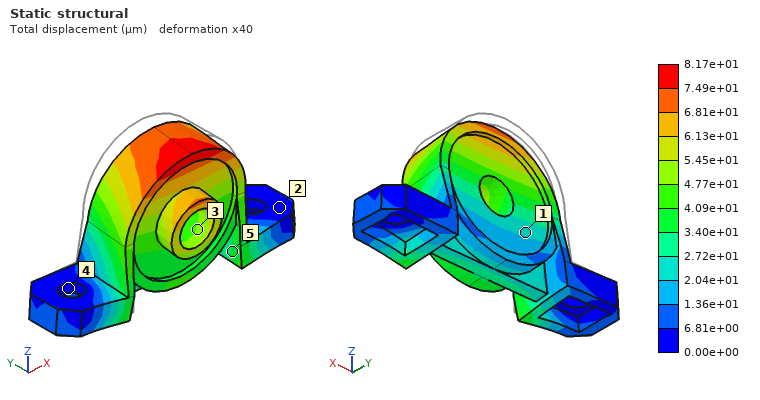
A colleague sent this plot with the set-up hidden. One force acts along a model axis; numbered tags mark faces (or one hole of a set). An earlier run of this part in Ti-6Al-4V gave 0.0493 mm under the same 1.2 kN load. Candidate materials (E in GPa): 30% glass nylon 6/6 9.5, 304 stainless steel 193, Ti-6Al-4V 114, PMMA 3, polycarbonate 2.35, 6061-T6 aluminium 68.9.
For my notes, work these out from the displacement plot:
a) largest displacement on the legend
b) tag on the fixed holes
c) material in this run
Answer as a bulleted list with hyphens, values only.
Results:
- 8.17e+01 µm
- 4
- 6061-T6 aluminium
